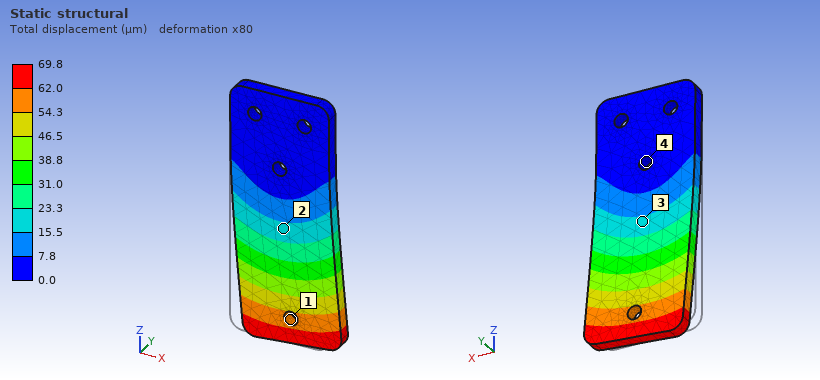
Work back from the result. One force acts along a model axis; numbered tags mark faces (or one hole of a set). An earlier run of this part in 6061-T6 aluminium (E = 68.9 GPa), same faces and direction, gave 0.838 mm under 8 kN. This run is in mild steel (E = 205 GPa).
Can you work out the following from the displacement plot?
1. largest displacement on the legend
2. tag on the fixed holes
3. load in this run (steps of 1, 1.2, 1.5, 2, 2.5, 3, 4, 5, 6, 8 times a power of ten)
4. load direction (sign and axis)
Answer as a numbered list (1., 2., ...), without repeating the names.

1. 69.8 µm
2. 4
3. 2 kN
4. +X
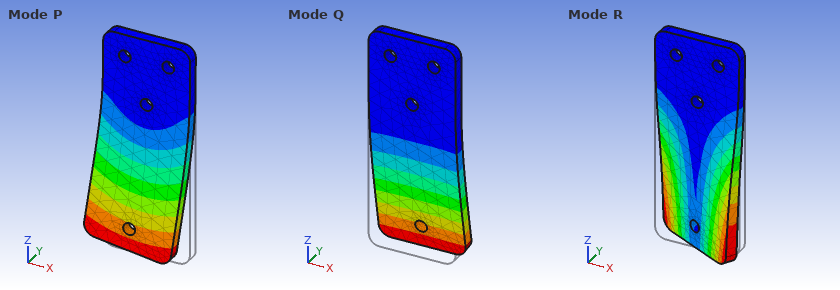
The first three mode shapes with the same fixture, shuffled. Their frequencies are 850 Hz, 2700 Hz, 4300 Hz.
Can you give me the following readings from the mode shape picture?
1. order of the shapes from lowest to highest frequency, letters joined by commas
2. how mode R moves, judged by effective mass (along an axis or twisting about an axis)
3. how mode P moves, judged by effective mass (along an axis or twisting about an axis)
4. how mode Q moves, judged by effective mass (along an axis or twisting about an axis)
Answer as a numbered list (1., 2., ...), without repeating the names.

1. Q, R, P
2. twisting about Z
3. along X
4. along Y
